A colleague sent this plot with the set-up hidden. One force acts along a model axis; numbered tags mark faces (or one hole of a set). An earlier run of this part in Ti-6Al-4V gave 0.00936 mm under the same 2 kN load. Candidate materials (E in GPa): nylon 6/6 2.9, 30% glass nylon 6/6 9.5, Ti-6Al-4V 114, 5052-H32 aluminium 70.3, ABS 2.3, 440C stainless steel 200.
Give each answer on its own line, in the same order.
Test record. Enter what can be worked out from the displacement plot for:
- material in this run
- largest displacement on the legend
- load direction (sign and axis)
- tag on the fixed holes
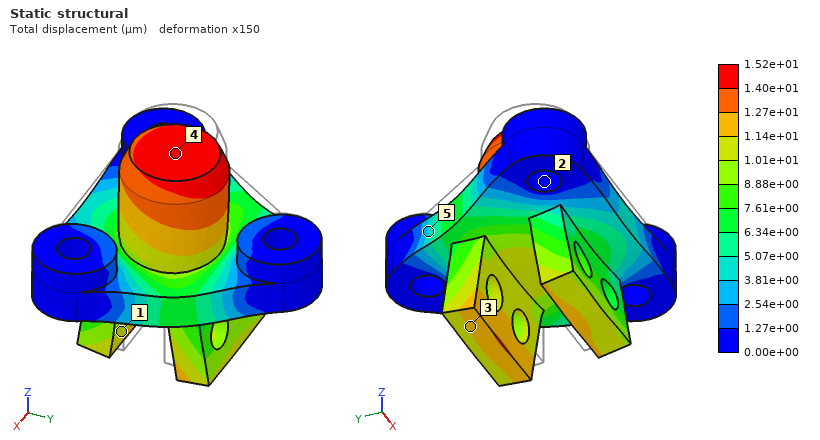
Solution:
5052-H32 aluminium
1.52e+01 µm
-Z
2
